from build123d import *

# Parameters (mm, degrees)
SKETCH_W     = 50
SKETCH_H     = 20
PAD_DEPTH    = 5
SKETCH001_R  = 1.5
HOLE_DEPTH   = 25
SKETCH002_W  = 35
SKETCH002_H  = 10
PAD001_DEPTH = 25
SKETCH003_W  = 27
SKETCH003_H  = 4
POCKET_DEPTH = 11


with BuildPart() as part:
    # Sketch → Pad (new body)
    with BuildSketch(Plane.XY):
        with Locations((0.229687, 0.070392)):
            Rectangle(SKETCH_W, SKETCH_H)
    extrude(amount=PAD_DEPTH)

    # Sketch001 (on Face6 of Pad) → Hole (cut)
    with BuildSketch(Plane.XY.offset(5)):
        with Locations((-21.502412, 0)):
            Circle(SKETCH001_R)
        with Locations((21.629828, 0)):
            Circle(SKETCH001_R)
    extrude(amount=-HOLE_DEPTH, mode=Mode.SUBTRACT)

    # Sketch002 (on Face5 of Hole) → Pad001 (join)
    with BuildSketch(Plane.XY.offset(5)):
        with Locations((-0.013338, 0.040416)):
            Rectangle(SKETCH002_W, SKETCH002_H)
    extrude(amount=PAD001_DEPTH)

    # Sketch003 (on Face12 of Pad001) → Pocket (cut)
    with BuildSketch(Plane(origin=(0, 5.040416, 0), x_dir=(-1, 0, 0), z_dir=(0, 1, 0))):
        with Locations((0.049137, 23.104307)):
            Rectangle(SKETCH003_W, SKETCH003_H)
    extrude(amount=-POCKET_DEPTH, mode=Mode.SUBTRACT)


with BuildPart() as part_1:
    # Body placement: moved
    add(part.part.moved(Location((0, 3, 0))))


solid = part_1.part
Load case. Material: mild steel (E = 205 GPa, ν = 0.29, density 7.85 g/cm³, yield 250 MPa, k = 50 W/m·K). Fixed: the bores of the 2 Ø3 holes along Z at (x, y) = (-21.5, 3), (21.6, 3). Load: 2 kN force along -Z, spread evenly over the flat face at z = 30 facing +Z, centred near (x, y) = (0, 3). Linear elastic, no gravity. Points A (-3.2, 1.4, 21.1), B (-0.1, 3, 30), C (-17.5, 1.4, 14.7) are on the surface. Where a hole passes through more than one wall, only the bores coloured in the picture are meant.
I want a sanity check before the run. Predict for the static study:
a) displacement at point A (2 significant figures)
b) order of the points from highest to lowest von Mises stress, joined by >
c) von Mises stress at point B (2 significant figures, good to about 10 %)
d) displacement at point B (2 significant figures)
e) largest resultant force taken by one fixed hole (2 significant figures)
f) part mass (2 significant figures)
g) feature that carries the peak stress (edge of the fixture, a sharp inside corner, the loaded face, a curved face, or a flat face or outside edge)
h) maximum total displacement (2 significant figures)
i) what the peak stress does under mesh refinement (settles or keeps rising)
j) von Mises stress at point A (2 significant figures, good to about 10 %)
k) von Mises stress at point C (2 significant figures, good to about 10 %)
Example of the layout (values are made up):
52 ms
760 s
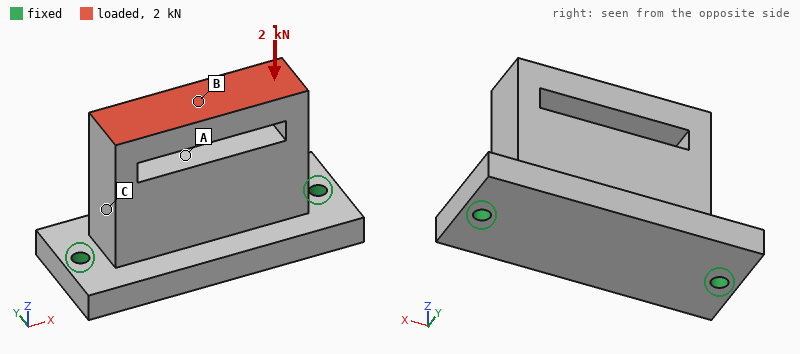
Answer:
2.7 µm
B > C > A
81 MPa
17 µm
1.0 kN
99 g
edge of the fixture
18 µm
keeps rising
10 MPa
28 MPa
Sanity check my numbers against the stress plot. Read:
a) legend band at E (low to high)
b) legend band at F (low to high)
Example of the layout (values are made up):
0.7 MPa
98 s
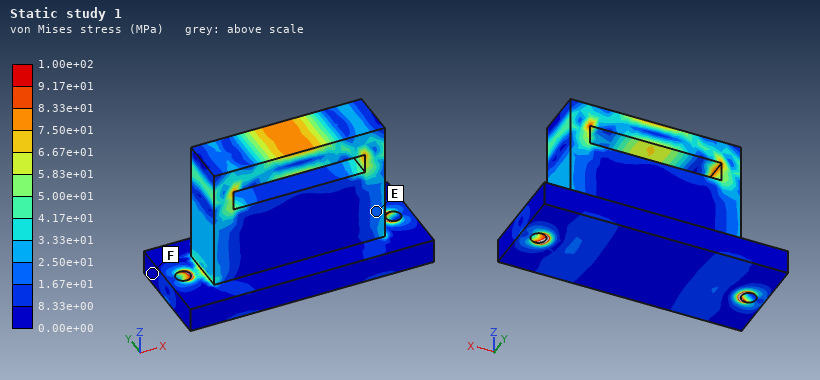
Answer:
1.67e+01 to 2.50e+01 MPa
0.00e+00 to 8.33e+00 MPa
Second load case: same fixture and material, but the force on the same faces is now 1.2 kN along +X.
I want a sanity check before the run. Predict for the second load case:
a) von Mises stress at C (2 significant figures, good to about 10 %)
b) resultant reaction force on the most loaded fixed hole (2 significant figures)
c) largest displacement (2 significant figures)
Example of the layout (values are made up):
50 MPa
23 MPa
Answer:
28 MPa
1.0 kN
13 µm
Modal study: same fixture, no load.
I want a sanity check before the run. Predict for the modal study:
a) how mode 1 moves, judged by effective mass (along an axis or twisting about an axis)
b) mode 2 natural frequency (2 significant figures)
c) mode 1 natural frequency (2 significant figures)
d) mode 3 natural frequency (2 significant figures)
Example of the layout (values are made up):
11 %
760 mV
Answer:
along Y
13 kHz
4100 Hz
13 kHz
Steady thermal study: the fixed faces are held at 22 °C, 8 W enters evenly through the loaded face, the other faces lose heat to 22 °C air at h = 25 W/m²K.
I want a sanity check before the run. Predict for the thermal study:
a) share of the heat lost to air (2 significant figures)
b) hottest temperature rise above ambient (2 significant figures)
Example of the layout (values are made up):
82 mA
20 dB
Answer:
19 %
39 K
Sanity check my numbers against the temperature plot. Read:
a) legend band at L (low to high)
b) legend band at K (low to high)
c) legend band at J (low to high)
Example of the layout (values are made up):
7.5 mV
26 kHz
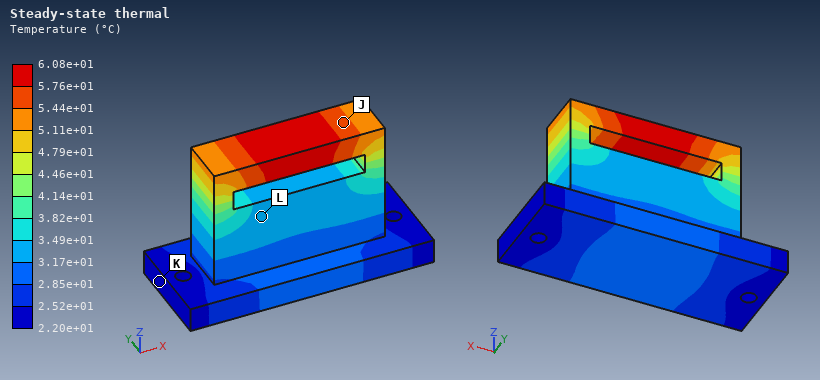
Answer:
3.17e+01 to 3.49e+01 °C
2.20e+01 to 2.52e+01 °C
5.44e+01 to 5.76e+01 °C
